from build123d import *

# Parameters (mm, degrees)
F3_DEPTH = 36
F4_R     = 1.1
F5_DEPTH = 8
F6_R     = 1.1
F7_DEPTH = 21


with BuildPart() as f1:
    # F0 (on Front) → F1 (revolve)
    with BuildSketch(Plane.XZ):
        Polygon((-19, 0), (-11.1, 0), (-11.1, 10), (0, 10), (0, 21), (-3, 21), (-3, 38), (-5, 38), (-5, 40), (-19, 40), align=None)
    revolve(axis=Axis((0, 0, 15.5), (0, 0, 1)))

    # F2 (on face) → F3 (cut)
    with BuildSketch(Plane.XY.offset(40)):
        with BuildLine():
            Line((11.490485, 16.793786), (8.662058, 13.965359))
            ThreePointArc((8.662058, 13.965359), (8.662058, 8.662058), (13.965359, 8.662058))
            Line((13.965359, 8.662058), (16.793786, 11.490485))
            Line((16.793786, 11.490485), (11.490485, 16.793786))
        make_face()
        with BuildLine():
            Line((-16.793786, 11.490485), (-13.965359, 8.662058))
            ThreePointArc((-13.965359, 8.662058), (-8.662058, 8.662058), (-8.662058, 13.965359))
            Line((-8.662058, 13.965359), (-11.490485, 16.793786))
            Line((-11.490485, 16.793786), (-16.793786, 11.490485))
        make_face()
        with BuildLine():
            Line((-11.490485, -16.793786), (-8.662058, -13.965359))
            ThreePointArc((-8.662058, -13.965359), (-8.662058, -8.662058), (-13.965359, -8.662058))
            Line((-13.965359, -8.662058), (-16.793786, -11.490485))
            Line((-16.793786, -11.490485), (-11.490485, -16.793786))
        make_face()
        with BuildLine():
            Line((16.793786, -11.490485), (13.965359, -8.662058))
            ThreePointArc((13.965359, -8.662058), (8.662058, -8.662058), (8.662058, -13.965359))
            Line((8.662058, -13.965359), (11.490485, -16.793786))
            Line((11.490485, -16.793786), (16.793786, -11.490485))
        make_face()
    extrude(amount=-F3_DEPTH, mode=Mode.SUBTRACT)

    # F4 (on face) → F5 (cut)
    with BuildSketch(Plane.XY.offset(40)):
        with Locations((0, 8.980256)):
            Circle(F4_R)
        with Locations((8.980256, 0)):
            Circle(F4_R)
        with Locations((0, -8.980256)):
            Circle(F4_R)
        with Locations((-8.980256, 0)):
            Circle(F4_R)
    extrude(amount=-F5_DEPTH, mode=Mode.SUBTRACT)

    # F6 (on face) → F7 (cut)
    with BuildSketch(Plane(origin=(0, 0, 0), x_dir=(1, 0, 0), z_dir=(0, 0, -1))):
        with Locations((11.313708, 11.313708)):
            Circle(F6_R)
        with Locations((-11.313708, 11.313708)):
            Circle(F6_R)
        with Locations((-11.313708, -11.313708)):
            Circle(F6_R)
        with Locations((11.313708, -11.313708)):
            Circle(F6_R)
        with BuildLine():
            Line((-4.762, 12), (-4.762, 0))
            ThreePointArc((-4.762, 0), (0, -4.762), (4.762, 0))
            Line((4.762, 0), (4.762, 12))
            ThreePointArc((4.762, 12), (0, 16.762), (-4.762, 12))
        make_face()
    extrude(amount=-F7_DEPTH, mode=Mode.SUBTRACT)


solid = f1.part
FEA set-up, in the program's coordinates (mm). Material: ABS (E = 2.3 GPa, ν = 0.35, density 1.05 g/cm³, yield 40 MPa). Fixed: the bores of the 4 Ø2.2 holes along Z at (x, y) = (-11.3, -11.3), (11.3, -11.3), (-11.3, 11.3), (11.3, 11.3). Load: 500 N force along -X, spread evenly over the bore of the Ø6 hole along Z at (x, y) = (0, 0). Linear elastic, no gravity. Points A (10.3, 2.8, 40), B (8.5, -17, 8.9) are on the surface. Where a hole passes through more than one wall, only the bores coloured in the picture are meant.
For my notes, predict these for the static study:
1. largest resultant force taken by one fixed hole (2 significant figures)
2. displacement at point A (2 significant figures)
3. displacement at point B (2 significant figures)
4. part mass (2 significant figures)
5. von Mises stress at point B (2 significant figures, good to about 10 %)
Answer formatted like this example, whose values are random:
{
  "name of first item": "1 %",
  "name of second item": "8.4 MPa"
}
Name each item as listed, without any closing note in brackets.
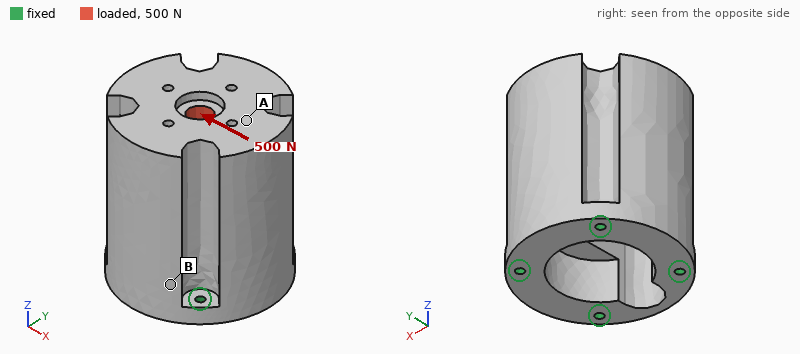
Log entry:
{
  "largest resultant force taken by one fixed hole": "350 N",
  "displacement at point A": "0.27 mm",
  "displacement at point B": "0.063 mm",
  "part mass": "33 g",
  "von Mises stress at point B": "4.5 MPa"
}
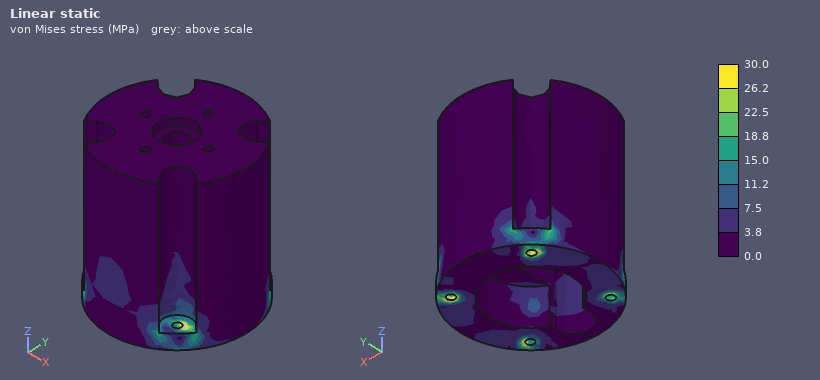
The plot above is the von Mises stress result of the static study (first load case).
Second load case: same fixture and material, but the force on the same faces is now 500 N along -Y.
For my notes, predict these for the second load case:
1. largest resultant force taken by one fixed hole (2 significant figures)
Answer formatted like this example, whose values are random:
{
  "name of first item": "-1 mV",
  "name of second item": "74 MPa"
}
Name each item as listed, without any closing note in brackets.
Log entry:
{
  "largest resultant force taken by one fixed hole": "320 N"
}
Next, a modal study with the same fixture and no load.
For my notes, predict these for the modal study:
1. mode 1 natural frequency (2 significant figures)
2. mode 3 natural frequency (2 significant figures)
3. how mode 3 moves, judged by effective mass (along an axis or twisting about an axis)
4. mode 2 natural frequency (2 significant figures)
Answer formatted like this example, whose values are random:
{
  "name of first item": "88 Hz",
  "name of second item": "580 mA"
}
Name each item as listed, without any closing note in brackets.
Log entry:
{
  "mode 1 natural frequency": "1600 Hz",
  "mode 3 natural frequency": "3900 Hz",
  "how mode 3 moves, judged by effective mass": "along Z",
  "mode 2 natural frequency": "1600 Hz"
}
